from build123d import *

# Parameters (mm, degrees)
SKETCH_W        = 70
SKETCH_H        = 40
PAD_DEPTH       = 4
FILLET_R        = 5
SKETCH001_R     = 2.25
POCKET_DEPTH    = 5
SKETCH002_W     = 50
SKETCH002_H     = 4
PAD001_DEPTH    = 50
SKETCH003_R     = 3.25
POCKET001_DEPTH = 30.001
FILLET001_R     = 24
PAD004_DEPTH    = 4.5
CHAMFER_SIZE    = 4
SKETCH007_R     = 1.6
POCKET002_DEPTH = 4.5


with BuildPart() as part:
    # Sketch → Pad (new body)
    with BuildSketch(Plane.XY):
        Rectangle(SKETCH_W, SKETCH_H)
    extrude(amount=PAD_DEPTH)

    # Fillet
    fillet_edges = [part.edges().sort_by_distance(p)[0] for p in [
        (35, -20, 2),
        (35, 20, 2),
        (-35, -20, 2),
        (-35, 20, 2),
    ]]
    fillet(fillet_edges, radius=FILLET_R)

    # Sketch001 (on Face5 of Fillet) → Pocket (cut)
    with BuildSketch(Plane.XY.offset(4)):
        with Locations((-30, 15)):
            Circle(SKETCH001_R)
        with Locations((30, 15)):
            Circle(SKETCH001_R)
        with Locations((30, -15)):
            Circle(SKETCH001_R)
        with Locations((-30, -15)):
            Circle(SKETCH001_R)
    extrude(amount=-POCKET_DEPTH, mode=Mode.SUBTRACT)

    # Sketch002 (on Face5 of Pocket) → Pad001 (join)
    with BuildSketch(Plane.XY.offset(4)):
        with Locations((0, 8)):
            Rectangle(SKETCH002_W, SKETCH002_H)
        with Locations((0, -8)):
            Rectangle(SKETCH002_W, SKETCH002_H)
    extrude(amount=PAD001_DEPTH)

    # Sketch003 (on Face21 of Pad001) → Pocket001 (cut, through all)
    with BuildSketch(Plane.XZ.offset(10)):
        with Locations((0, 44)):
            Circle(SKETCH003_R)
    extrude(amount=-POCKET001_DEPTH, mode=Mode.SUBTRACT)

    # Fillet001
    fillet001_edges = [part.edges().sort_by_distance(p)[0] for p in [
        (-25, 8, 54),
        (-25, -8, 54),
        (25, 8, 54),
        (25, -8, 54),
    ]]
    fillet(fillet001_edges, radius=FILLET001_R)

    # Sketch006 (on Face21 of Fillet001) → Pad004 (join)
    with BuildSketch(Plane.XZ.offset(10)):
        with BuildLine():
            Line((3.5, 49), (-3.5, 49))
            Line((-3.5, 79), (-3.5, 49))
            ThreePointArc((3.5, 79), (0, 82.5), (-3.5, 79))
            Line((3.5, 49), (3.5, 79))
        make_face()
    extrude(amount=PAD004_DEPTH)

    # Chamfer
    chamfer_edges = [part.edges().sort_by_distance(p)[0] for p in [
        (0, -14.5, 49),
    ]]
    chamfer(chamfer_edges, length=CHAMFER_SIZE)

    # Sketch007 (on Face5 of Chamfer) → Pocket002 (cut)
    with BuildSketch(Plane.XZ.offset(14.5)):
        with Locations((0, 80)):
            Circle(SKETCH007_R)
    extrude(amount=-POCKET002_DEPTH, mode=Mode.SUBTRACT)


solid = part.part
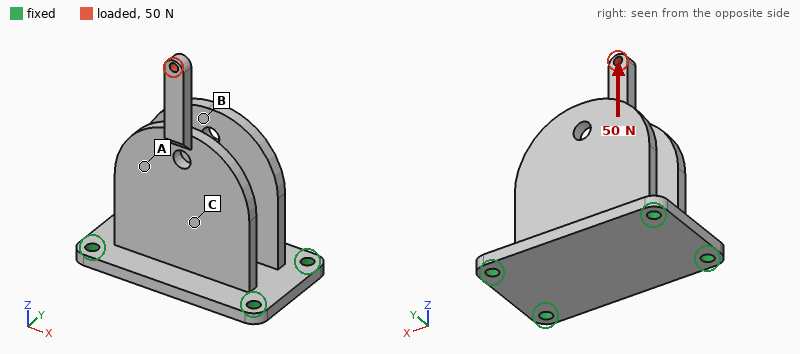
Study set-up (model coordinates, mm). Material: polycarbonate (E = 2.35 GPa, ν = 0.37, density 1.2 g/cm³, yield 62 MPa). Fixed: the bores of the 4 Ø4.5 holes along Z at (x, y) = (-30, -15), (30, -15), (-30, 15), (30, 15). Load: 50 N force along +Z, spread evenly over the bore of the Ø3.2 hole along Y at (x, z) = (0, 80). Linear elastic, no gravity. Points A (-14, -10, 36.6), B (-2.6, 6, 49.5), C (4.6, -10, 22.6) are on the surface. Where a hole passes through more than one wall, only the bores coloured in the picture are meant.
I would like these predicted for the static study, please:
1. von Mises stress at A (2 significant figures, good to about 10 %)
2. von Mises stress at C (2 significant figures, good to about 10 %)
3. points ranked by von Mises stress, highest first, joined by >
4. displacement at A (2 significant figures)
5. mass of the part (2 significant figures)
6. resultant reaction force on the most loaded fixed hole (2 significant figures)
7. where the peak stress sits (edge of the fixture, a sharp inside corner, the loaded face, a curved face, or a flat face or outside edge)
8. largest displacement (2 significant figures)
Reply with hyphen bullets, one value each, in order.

- 2.0 MPa
- 1.6 MPa
- A > C > B
- 0.22 mm
- 35 g
- 25 N
- a flat face or outside edge
- 1.3 mm
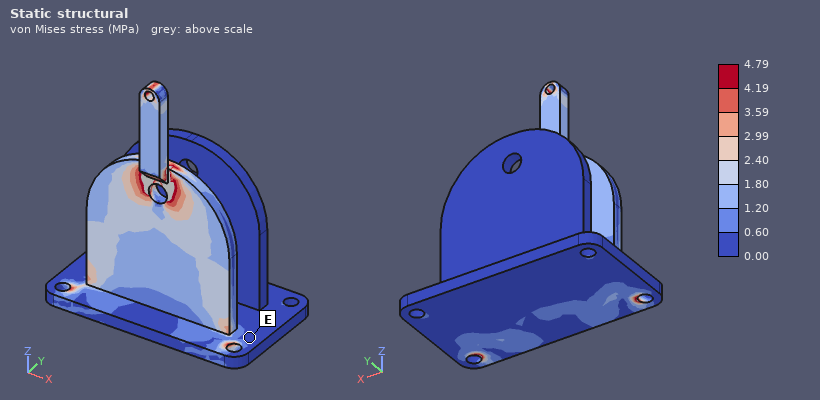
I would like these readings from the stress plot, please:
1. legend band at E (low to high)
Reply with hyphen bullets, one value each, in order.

- 0.00 to 0.60 MPa
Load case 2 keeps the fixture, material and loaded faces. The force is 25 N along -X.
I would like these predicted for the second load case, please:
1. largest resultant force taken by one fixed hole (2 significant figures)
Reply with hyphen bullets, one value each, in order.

- 31 N
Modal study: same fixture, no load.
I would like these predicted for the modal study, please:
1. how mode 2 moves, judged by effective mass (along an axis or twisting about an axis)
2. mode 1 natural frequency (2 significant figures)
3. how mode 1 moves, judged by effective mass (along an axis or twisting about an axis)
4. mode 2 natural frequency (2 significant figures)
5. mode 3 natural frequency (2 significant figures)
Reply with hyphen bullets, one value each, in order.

- along Y
- 270 Hz
- along Y
- 380 Hz
- 880 Hz
